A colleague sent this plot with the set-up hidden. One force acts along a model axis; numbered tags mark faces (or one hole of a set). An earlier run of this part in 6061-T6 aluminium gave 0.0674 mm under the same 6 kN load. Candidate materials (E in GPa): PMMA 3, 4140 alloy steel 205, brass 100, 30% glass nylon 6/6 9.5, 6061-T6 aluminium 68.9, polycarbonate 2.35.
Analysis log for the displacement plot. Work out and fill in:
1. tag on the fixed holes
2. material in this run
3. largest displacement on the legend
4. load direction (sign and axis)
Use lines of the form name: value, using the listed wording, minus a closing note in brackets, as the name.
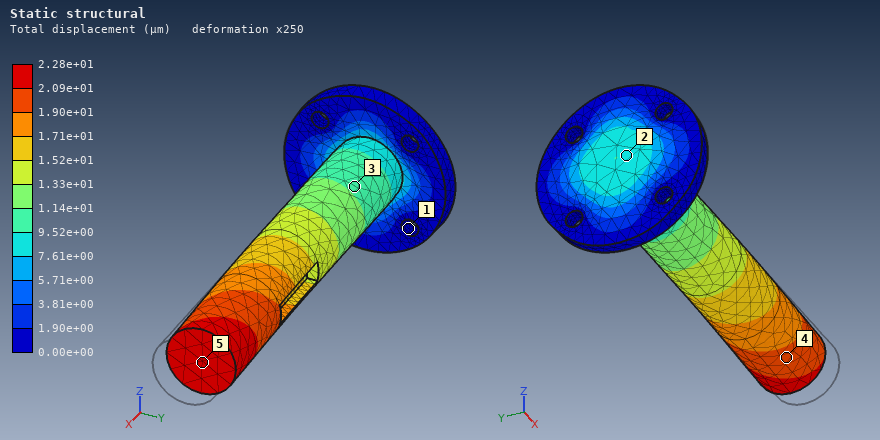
tag on the fixed holes: 1
material in this run: 4140 alloy steel
largest displacement on the legend: 2.28e+01 µm
load direction: -X
